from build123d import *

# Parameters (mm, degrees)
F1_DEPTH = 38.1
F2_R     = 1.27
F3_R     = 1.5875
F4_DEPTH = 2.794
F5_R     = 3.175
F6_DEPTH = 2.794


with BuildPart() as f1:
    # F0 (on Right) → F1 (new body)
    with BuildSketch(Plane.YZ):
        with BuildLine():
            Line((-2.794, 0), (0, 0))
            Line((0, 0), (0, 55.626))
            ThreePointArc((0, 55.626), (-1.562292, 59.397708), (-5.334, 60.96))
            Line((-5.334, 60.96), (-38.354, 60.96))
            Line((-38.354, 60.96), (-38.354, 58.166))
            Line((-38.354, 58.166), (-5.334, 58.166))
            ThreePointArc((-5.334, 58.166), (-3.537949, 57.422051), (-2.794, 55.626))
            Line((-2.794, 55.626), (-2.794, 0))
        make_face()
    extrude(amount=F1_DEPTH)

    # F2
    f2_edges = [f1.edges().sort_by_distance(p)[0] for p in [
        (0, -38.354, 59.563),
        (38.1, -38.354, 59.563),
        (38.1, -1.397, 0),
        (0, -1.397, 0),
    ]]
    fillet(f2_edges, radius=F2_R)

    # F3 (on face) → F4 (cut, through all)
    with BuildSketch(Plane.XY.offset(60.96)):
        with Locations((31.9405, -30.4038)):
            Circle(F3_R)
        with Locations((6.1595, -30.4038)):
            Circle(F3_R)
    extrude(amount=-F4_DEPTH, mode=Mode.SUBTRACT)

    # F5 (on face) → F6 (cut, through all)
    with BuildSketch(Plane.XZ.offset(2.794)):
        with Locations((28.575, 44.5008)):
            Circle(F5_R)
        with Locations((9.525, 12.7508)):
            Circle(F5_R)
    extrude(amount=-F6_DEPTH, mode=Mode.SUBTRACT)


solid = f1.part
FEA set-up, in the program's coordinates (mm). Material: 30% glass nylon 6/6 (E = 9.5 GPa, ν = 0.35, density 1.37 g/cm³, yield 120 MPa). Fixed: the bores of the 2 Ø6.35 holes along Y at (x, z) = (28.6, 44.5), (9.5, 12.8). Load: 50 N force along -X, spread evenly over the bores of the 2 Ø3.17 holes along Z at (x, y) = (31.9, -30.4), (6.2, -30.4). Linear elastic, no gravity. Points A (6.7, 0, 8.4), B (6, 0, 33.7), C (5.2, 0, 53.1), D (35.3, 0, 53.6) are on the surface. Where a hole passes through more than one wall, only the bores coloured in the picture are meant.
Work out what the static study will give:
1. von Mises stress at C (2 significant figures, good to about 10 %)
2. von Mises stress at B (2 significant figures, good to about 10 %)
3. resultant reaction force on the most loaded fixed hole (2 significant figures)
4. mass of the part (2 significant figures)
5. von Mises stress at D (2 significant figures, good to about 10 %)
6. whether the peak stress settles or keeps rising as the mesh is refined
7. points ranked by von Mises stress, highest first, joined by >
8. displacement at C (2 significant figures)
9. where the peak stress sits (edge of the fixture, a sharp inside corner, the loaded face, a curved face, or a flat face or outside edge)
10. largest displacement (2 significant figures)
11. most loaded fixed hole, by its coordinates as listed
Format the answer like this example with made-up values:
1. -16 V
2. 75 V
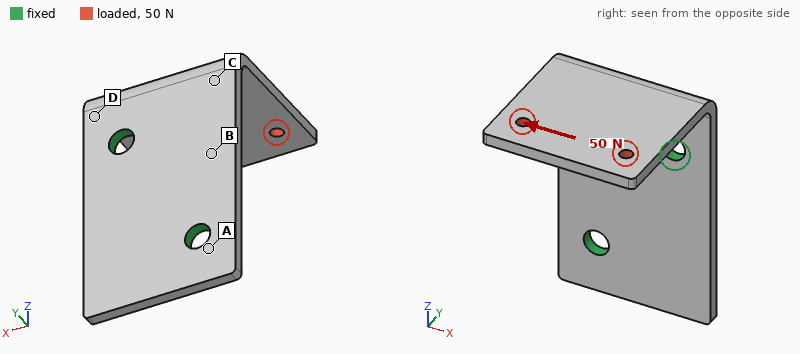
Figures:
1. 6.6 MPa
2. 9.4 MPa
3. 59 N
4. 14 g
5. 18 MPa
6. keeps rising
7. D > B > C > A
8. 0.32 mm
9. edge of the fixture
10. 0.87 mm
11. (28.6, 44.5)
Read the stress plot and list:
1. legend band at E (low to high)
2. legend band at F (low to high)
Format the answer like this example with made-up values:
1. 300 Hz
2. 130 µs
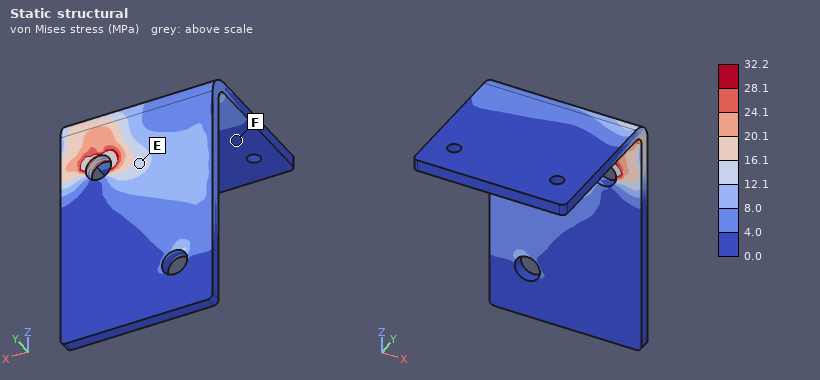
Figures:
1. 12.1 to 16.1 MPa
2. 0.0 to 4.0 MPa
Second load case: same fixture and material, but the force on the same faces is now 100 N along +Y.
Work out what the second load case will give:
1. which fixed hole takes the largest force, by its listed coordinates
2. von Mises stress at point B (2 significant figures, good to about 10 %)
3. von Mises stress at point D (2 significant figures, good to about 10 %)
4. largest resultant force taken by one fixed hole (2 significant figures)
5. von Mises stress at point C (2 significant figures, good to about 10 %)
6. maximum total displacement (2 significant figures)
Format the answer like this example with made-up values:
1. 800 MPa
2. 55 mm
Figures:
1. (28.6, 44.5)
2. 8.2 MPa
3. 20 MPa
4. 110 N
5. 6.7 MPa
6. 0.95 mm
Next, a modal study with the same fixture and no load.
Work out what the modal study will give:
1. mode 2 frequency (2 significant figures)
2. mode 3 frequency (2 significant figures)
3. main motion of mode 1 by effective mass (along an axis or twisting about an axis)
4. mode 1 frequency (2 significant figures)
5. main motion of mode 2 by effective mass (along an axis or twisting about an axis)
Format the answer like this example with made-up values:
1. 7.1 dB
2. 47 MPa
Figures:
1. 790 Hz
2. 1800 Hz
3. along Z
4. 540 Hz
5. along X
